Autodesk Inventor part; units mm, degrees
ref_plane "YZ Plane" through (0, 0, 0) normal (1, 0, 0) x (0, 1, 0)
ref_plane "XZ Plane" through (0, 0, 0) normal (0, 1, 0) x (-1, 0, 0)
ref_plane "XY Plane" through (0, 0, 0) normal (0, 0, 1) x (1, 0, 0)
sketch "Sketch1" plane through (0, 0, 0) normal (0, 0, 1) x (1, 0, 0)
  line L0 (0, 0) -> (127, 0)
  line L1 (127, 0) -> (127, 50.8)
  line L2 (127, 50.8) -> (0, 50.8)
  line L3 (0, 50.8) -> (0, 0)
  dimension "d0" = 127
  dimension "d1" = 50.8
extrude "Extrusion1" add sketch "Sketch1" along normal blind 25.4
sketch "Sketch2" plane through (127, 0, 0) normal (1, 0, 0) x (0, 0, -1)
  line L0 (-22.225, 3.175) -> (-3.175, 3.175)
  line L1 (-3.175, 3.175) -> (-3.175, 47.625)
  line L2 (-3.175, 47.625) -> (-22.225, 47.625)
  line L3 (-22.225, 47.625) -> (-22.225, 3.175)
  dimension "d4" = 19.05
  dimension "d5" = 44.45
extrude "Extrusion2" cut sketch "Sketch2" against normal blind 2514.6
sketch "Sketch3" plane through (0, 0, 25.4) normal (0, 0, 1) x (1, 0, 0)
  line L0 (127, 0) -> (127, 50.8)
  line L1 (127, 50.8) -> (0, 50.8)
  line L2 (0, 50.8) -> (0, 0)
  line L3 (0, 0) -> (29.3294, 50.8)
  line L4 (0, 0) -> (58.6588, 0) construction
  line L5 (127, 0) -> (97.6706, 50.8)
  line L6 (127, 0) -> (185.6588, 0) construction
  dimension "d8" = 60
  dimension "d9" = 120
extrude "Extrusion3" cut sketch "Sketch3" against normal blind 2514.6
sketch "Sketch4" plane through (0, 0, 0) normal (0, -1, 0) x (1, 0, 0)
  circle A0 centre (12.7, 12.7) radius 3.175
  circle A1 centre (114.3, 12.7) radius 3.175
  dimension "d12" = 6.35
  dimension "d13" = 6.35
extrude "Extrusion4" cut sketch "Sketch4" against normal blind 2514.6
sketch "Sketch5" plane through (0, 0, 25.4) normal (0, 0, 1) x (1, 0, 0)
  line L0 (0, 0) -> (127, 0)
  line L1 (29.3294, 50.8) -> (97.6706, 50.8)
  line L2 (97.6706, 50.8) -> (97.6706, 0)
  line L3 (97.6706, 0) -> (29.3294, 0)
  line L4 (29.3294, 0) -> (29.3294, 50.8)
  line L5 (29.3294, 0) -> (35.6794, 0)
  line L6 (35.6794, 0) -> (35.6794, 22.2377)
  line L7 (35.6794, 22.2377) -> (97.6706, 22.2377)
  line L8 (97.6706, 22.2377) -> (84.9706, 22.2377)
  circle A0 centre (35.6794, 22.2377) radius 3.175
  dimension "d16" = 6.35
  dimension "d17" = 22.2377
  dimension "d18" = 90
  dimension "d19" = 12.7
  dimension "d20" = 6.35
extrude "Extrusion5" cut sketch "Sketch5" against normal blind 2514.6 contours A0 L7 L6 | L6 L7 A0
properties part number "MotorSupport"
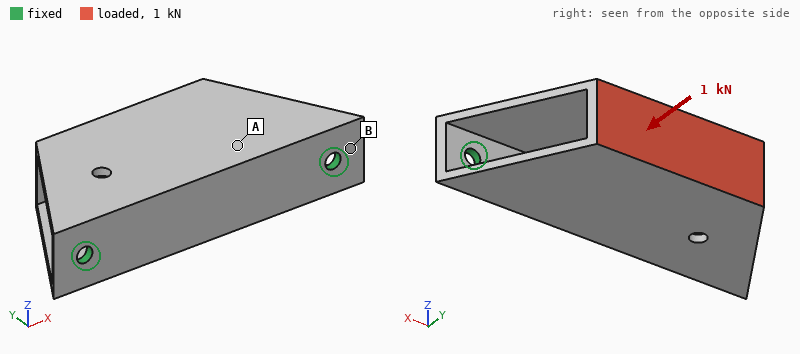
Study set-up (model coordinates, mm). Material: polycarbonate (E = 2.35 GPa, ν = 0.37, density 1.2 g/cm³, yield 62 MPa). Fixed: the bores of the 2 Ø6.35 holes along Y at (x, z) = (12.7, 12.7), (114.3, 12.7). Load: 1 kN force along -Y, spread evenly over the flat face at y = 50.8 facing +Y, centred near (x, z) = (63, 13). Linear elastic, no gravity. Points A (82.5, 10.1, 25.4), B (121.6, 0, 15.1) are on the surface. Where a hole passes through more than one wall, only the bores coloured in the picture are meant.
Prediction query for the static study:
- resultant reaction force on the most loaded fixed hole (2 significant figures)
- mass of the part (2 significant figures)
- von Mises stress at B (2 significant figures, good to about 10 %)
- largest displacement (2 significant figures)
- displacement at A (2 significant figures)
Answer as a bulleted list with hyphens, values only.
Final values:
- 560 N
- 52 g
- 22 MPa
- 0.65 mm
- 0.46 mm
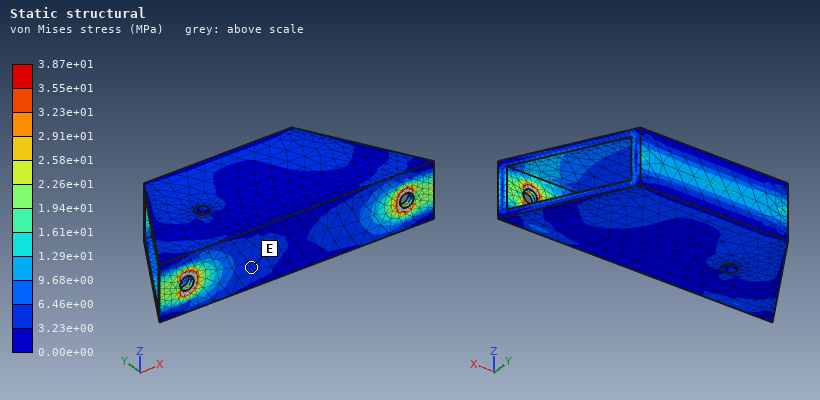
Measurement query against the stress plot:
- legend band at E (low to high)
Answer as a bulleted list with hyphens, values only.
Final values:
- 3.23e+00 to 6.46e+00 MPa
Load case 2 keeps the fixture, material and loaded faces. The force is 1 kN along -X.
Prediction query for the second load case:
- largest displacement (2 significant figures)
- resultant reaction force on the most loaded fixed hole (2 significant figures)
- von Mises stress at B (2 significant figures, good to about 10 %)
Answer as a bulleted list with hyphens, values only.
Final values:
- 0.61 mm
- 700 N
- 25 MPa
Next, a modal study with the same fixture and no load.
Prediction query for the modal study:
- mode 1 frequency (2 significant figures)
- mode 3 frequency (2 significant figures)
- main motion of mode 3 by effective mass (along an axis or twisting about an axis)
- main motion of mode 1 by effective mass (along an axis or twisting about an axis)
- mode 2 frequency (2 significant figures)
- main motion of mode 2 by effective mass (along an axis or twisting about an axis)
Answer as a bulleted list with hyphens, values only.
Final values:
- 240 Hz
- 1100 Hz
- twisting about Y
- along Z
- 1100 Hz
- along Y
